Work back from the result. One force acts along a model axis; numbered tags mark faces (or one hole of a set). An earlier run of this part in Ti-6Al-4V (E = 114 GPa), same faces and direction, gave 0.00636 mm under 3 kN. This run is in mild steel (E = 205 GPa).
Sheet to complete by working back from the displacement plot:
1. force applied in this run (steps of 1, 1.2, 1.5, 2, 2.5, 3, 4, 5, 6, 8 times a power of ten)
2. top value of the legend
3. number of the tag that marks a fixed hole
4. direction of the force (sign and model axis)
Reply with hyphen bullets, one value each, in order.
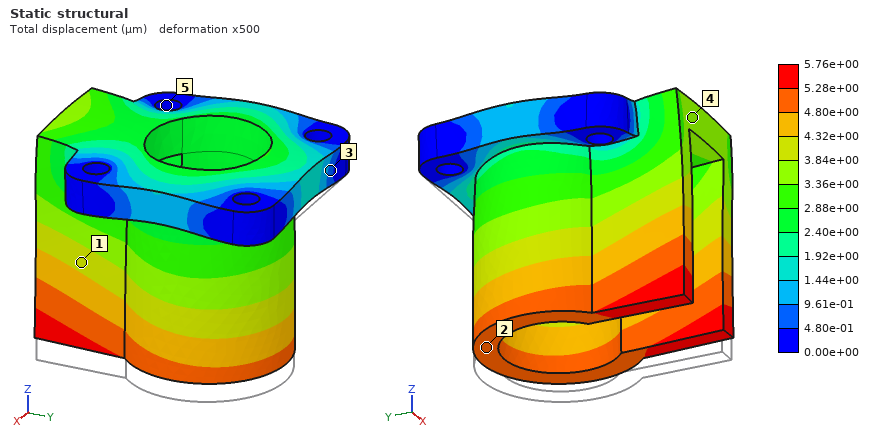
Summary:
- 5 kN
- 5.76e+00 µm
- 5
- +Z
